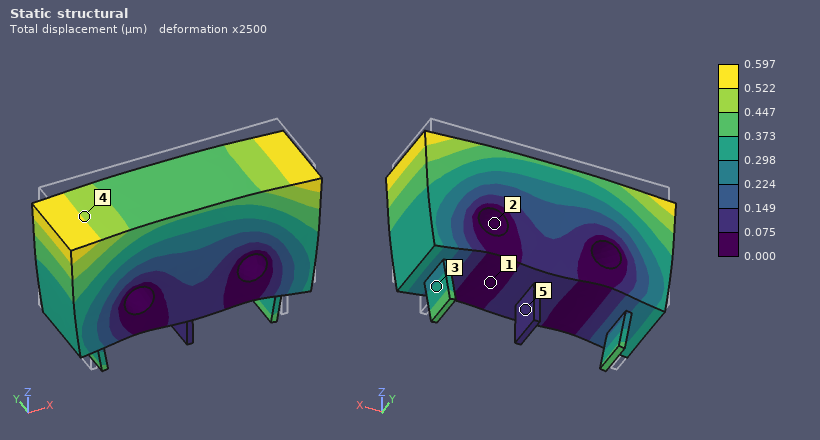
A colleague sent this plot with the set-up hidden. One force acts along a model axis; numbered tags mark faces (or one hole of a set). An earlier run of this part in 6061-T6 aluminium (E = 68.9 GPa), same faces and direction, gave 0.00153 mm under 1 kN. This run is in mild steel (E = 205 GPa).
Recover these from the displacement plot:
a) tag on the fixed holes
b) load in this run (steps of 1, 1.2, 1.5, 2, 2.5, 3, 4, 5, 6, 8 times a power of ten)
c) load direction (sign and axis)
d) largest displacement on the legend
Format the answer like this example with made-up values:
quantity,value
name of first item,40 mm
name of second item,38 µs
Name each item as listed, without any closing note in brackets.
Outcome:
quantity,value
tag on the fixed holes,2
load in this run,1.2 kN
load direction,-Z
largest displacement on the legend,0.597 µm
